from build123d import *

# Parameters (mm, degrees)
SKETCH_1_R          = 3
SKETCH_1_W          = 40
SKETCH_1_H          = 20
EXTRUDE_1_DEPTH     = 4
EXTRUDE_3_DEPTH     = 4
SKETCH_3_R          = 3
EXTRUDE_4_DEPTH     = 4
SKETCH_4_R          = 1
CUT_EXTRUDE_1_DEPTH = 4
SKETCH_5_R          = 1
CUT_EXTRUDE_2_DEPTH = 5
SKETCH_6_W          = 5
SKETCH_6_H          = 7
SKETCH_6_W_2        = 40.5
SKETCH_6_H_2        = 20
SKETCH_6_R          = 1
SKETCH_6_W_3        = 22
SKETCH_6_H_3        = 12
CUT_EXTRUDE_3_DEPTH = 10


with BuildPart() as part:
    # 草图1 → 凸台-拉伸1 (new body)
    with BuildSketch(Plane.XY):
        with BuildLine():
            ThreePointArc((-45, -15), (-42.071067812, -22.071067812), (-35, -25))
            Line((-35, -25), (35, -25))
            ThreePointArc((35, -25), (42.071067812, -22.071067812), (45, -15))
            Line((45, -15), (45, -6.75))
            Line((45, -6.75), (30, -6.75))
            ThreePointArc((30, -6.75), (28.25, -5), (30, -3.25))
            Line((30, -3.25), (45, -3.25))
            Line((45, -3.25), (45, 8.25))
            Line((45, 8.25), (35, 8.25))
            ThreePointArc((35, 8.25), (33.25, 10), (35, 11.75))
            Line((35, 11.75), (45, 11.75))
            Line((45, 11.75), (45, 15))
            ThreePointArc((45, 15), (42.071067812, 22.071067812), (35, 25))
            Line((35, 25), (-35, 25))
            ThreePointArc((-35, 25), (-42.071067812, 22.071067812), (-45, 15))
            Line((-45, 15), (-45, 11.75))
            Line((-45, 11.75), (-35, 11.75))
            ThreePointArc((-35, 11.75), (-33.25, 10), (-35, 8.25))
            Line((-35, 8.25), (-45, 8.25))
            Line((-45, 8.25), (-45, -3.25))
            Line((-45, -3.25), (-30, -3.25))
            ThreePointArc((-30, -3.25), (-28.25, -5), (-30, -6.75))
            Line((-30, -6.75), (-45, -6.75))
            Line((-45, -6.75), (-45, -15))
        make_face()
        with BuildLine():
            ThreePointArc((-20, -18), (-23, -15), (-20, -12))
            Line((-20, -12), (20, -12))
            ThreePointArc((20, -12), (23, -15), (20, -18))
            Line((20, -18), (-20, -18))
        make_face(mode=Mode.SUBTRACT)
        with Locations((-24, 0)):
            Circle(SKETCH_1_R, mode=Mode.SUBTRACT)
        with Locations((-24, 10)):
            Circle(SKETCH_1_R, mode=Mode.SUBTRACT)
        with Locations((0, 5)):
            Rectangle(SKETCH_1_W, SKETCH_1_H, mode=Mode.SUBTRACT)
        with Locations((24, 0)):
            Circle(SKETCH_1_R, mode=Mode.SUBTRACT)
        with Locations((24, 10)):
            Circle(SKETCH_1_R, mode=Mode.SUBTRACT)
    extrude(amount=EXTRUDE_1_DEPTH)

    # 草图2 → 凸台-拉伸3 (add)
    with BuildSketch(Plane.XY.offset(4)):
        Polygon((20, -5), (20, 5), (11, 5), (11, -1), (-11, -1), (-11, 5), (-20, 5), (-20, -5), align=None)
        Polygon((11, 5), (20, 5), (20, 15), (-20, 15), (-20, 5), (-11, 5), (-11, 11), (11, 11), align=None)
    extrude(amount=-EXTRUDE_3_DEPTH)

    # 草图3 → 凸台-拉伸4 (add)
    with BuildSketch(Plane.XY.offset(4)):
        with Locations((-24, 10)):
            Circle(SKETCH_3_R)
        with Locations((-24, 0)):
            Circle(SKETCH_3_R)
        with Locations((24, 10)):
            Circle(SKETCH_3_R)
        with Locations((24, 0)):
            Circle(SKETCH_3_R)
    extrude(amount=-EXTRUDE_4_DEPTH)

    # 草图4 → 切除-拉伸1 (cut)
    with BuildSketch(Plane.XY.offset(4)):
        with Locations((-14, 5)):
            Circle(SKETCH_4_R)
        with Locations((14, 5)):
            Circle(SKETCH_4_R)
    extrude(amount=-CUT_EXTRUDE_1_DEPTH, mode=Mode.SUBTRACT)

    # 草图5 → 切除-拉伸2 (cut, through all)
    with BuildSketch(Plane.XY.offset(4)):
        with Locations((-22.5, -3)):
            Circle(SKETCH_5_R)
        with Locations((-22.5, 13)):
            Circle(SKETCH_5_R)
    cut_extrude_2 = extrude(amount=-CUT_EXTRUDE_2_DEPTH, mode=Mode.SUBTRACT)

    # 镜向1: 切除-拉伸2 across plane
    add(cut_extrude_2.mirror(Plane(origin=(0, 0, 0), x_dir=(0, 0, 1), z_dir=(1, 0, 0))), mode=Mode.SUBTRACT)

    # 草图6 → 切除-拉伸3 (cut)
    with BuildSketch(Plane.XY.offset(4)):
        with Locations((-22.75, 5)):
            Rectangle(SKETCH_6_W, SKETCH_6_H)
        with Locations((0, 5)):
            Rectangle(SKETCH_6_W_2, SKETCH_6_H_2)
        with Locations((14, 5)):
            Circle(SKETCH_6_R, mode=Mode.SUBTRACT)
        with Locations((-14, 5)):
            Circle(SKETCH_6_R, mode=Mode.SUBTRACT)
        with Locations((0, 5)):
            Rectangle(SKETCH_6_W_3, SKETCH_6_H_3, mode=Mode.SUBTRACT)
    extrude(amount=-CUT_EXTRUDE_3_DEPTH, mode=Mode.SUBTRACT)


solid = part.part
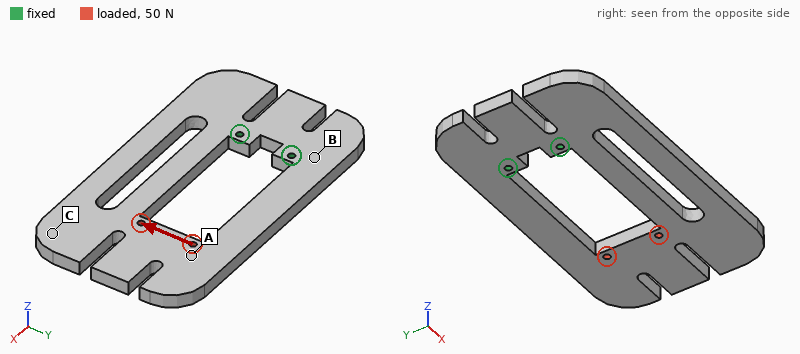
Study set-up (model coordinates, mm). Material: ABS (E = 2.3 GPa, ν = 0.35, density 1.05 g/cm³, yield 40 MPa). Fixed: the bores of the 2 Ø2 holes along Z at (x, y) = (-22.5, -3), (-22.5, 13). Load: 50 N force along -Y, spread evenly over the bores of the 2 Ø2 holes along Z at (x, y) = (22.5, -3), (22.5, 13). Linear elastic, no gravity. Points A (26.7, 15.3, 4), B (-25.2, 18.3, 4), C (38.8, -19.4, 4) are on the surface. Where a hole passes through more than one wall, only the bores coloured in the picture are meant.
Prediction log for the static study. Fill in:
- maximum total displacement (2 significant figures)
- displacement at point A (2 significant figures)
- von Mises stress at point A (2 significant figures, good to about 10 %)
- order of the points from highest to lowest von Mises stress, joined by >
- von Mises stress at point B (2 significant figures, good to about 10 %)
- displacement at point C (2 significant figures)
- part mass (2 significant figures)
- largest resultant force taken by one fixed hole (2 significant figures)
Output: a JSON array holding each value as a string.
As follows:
["1.1 mm", "0.89 mm", "3.0 MPa", "B > A > C", "5.2 MPa", "1.1 mm", "13 g", "120 N"]
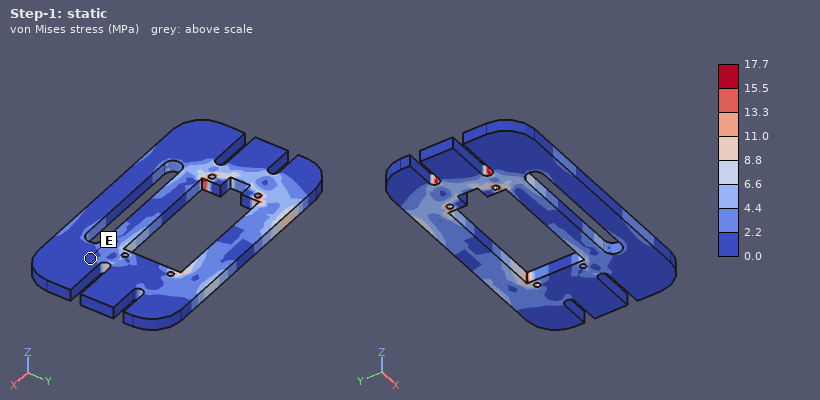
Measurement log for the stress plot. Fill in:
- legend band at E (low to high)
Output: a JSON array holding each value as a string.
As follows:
["0.0 to 2.2 MPa"]
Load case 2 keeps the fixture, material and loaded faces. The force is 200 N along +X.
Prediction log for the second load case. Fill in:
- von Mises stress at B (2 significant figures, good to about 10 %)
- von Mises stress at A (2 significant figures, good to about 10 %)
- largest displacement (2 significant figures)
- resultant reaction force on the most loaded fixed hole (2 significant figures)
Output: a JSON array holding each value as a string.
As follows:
["2.6 MPa", "3.2 MPa", "0.17 mm", "110 N"]
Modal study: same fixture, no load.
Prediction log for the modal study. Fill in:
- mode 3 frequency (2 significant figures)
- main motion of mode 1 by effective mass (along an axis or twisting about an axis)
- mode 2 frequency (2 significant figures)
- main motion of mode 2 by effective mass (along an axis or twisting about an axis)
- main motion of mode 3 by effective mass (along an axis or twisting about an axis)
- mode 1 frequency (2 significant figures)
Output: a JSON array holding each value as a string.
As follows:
["450 Hz", "along Z", "380 Hz", "twisting about X", "along Y", "140 Hz"]
